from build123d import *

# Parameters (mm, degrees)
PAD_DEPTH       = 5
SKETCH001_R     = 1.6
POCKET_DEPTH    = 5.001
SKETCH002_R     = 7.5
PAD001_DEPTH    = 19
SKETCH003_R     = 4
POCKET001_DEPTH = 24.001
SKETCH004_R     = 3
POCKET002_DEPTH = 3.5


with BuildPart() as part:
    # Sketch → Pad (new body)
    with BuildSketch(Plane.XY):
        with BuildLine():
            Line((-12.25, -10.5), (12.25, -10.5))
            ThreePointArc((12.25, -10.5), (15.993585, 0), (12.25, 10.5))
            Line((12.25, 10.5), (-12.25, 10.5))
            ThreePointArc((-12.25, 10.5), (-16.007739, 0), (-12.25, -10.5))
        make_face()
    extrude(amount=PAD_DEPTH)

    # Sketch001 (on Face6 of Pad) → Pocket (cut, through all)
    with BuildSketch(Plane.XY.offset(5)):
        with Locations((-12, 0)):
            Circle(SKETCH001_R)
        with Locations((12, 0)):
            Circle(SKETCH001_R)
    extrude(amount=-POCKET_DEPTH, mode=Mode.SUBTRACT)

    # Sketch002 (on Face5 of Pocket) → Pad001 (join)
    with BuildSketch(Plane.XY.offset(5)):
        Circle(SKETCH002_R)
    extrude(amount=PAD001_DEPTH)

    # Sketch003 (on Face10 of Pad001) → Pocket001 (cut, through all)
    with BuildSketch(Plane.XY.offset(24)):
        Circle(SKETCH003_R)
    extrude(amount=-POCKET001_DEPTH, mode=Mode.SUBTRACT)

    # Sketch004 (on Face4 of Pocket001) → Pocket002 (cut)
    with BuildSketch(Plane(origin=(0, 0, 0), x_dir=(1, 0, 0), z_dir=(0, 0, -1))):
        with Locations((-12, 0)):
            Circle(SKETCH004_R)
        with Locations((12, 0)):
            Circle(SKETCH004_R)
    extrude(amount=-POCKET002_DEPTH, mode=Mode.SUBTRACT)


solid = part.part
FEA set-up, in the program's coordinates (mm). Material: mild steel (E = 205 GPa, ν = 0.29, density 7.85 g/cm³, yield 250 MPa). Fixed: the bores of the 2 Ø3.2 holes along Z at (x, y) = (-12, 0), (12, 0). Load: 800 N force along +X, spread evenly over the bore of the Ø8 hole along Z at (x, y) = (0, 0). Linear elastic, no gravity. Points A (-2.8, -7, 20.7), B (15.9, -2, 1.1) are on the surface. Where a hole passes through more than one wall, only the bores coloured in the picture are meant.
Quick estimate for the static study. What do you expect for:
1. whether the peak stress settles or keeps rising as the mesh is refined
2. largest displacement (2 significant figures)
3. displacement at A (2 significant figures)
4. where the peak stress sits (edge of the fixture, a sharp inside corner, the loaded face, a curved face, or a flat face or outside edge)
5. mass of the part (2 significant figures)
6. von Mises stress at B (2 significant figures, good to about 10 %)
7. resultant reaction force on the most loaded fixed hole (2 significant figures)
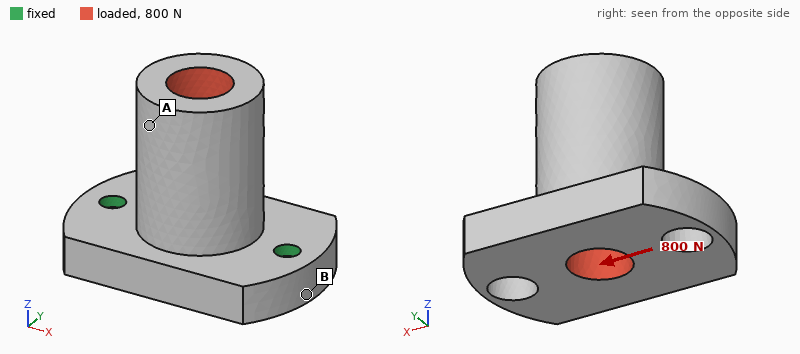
keeps rising
7.0 µm
5.7 µm
edge of the fixture
40 g
12 MPa
490 N
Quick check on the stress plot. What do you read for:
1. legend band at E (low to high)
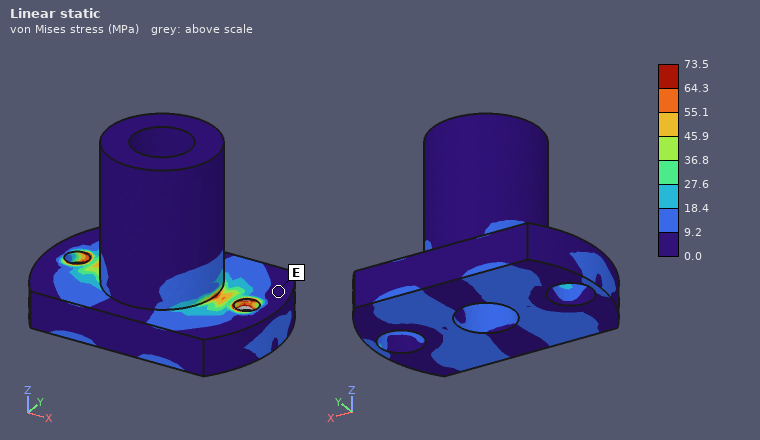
0.0 to 9.2 MPa
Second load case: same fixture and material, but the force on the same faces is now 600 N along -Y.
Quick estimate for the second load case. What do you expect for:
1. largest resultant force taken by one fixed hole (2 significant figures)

300 N
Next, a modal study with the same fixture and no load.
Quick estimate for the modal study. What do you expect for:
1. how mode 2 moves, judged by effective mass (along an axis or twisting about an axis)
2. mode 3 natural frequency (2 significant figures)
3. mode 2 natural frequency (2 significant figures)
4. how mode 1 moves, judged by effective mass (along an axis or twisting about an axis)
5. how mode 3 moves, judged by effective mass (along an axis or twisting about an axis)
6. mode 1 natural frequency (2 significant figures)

along X
15 kHz
13 kHz
along Y
along Z
4200 Hz
